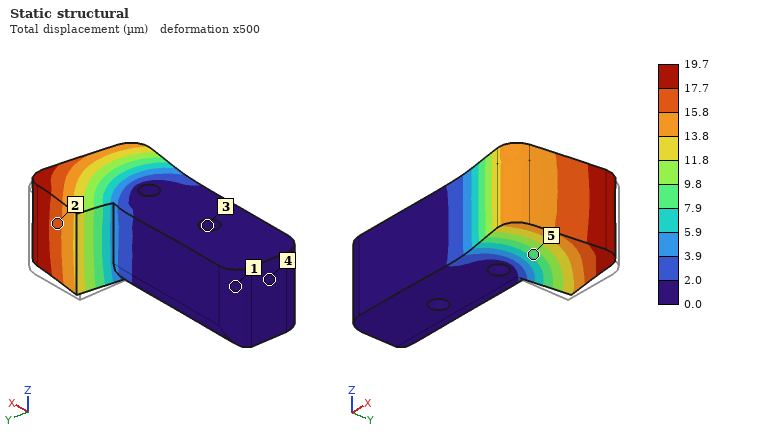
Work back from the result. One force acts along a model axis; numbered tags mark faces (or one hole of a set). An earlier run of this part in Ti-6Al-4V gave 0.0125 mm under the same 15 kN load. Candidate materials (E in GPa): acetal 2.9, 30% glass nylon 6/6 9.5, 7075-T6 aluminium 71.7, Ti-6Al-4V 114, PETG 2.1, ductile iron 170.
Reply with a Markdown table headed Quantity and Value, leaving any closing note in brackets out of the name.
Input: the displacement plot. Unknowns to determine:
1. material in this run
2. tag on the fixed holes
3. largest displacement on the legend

| Quantity | Value |
|---|---|
| material in this run | 7075-T6 aluminium |
| tag on the fixed holes | 3 |
| largest displacement on the legend | 19.7 µm |
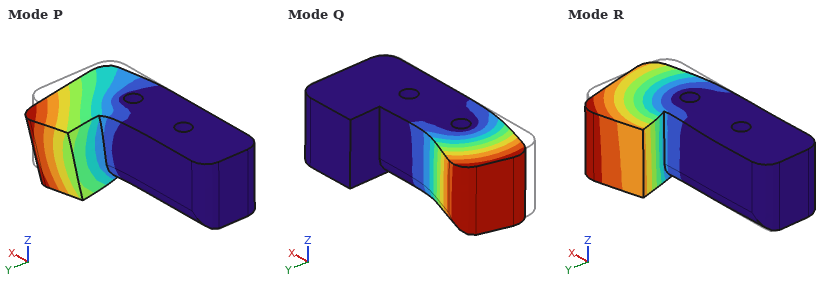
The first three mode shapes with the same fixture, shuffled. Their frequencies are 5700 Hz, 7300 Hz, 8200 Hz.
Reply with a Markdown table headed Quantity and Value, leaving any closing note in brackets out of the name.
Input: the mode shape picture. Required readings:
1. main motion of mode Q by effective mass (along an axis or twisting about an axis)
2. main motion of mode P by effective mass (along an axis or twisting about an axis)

| Quantity | Value |
|---|---|
| main motion of mode Q by effective mass | along Y |
| main motion of mode P by effective mass | along Z |
